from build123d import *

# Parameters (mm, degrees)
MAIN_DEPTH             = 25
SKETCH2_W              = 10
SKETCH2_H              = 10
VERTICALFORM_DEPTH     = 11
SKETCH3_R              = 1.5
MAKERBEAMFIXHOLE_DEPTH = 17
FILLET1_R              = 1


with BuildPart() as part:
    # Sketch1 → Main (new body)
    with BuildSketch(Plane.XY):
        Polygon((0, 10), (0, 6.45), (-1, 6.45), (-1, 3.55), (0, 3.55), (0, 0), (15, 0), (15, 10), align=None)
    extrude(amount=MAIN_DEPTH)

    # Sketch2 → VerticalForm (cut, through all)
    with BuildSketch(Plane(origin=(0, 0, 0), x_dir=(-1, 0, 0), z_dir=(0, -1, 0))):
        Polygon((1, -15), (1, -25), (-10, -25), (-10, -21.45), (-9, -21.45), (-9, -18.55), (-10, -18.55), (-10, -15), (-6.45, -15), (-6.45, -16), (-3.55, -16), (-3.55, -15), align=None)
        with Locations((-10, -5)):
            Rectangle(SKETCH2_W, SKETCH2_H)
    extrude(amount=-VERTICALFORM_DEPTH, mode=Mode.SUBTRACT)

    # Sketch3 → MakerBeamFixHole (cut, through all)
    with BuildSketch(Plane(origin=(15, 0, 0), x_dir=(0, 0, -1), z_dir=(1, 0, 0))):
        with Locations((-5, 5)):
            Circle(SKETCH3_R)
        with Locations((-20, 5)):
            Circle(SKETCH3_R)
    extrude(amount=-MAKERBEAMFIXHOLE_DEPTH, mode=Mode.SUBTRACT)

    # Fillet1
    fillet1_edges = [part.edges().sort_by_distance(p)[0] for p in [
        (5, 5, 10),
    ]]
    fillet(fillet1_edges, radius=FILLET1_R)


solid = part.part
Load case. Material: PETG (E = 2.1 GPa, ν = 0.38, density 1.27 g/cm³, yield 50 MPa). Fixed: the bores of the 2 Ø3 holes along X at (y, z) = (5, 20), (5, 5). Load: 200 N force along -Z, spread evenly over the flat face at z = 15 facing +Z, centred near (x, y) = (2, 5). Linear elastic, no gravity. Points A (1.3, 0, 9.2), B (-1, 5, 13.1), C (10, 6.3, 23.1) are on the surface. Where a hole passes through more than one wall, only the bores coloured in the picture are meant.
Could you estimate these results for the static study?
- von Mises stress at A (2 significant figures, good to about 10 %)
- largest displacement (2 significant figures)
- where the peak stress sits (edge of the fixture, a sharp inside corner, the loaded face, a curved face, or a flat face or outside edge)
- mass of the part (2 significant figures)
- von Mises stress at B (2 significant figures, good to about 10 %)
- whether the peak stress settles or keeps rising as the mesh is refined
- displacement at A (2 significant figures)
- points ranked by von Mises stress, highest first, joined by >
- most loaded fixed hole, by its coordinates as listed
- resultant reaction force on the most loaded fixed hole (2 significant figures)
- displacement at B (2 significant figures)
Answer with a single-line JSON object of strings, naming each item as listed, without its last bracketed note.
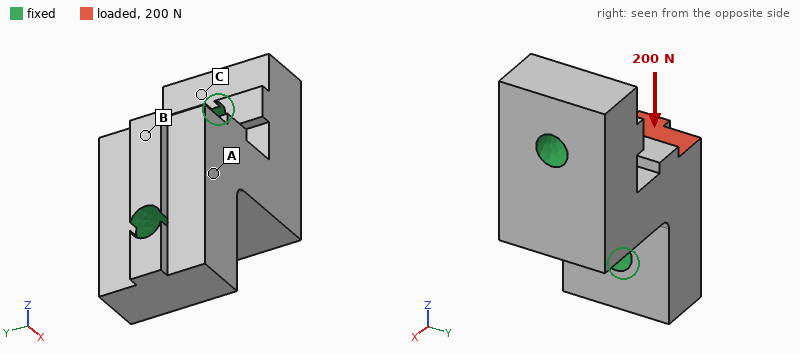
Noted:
{"von Mises stress at A": "3.2 MPa", "largest displacement": "28 µm", "where the peak stress sits": "edge of the fixture", "mass of the part": "2.2 g", "von Mises stress at B": "6.0 MPa", "whether the peak stress settles or keeps rising as the mesh is refined": "keeps rising", "displacement at A": "12 µm", "points ranked by von Mises stress, highest first, joined by >": "B > A > C", "most loaded fixed hole, by its coordinates as listed": "(5, 5)", "resultant reaction force on the most loaded fixed hole": "200 N", "displacement at B": "22 µm"}
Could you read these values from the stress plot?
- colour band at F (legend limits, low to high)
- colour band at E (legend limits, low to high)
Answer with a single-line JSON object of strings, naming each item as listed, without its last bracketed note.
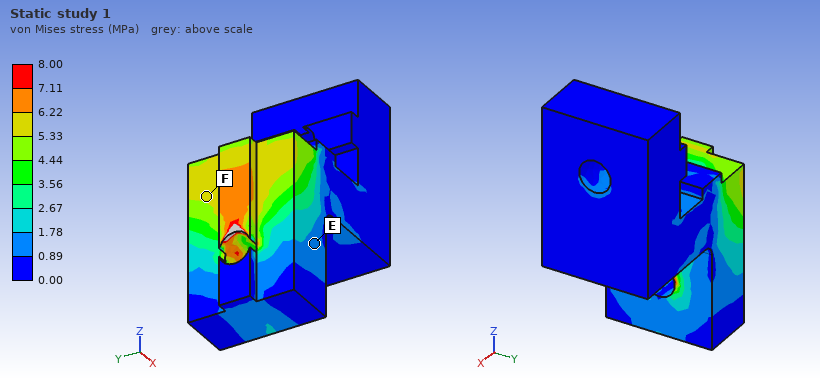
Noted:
{"colour band at F": "5.33 to 6.22 MPa", "colour band at E": "0.89 to 1.78 MPa"}
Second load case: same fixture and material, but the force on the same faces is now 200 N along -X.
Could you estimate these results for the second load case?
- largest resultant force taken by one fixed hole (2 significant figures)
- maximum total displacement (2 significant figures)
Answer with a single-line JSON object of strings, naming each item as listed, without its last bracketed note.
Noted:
{"largest resultant force taken by one fixed hole": "110 N", "maximum total displacement": "97 µm"}
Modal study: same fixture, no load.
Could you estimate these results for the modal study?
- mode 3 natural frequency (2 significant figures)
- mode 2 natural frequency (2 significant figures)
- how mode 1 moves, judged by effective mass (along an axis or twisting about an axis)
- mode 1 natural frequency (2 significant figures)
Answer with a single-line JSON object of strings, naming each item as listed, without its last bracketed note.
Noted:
{"mode 3 natural frequency": "11 kHz", "mode 2 natural frequency": "10 kHz", "how mode 1 moves, judged by effective mass": "along Y", "mode 1 natural frequency": "9800 Hz"}
